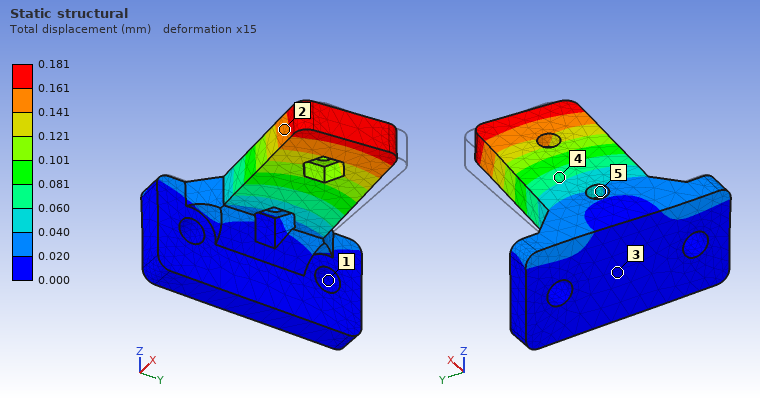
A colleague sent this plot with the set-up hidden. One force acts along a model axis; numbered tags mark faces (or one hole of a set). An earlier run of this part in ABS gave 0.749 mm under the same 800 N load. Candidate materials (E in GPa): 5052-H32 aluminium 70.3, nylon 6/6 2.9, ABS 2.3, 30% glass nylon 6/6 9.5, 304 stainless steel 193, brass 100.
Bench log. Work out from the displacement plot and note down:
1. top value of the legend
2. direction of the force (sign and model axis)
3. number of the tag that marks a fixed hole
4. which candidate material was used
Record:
0.181 mm
-Y
1
30% glass nylon 6/6
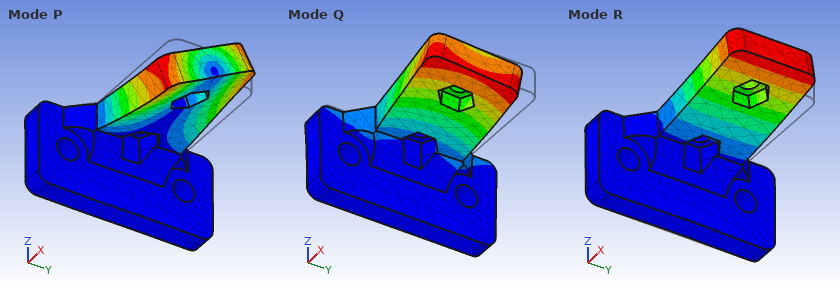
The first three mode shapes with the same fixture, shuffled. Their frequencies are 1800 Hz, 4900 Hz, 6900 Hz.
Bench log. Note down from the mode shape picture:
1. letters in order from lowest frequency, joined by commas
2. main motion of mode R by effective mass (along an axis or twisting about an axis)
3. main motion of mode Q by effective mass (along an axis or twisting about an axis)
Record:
R, Q, P
along Z
along Y
